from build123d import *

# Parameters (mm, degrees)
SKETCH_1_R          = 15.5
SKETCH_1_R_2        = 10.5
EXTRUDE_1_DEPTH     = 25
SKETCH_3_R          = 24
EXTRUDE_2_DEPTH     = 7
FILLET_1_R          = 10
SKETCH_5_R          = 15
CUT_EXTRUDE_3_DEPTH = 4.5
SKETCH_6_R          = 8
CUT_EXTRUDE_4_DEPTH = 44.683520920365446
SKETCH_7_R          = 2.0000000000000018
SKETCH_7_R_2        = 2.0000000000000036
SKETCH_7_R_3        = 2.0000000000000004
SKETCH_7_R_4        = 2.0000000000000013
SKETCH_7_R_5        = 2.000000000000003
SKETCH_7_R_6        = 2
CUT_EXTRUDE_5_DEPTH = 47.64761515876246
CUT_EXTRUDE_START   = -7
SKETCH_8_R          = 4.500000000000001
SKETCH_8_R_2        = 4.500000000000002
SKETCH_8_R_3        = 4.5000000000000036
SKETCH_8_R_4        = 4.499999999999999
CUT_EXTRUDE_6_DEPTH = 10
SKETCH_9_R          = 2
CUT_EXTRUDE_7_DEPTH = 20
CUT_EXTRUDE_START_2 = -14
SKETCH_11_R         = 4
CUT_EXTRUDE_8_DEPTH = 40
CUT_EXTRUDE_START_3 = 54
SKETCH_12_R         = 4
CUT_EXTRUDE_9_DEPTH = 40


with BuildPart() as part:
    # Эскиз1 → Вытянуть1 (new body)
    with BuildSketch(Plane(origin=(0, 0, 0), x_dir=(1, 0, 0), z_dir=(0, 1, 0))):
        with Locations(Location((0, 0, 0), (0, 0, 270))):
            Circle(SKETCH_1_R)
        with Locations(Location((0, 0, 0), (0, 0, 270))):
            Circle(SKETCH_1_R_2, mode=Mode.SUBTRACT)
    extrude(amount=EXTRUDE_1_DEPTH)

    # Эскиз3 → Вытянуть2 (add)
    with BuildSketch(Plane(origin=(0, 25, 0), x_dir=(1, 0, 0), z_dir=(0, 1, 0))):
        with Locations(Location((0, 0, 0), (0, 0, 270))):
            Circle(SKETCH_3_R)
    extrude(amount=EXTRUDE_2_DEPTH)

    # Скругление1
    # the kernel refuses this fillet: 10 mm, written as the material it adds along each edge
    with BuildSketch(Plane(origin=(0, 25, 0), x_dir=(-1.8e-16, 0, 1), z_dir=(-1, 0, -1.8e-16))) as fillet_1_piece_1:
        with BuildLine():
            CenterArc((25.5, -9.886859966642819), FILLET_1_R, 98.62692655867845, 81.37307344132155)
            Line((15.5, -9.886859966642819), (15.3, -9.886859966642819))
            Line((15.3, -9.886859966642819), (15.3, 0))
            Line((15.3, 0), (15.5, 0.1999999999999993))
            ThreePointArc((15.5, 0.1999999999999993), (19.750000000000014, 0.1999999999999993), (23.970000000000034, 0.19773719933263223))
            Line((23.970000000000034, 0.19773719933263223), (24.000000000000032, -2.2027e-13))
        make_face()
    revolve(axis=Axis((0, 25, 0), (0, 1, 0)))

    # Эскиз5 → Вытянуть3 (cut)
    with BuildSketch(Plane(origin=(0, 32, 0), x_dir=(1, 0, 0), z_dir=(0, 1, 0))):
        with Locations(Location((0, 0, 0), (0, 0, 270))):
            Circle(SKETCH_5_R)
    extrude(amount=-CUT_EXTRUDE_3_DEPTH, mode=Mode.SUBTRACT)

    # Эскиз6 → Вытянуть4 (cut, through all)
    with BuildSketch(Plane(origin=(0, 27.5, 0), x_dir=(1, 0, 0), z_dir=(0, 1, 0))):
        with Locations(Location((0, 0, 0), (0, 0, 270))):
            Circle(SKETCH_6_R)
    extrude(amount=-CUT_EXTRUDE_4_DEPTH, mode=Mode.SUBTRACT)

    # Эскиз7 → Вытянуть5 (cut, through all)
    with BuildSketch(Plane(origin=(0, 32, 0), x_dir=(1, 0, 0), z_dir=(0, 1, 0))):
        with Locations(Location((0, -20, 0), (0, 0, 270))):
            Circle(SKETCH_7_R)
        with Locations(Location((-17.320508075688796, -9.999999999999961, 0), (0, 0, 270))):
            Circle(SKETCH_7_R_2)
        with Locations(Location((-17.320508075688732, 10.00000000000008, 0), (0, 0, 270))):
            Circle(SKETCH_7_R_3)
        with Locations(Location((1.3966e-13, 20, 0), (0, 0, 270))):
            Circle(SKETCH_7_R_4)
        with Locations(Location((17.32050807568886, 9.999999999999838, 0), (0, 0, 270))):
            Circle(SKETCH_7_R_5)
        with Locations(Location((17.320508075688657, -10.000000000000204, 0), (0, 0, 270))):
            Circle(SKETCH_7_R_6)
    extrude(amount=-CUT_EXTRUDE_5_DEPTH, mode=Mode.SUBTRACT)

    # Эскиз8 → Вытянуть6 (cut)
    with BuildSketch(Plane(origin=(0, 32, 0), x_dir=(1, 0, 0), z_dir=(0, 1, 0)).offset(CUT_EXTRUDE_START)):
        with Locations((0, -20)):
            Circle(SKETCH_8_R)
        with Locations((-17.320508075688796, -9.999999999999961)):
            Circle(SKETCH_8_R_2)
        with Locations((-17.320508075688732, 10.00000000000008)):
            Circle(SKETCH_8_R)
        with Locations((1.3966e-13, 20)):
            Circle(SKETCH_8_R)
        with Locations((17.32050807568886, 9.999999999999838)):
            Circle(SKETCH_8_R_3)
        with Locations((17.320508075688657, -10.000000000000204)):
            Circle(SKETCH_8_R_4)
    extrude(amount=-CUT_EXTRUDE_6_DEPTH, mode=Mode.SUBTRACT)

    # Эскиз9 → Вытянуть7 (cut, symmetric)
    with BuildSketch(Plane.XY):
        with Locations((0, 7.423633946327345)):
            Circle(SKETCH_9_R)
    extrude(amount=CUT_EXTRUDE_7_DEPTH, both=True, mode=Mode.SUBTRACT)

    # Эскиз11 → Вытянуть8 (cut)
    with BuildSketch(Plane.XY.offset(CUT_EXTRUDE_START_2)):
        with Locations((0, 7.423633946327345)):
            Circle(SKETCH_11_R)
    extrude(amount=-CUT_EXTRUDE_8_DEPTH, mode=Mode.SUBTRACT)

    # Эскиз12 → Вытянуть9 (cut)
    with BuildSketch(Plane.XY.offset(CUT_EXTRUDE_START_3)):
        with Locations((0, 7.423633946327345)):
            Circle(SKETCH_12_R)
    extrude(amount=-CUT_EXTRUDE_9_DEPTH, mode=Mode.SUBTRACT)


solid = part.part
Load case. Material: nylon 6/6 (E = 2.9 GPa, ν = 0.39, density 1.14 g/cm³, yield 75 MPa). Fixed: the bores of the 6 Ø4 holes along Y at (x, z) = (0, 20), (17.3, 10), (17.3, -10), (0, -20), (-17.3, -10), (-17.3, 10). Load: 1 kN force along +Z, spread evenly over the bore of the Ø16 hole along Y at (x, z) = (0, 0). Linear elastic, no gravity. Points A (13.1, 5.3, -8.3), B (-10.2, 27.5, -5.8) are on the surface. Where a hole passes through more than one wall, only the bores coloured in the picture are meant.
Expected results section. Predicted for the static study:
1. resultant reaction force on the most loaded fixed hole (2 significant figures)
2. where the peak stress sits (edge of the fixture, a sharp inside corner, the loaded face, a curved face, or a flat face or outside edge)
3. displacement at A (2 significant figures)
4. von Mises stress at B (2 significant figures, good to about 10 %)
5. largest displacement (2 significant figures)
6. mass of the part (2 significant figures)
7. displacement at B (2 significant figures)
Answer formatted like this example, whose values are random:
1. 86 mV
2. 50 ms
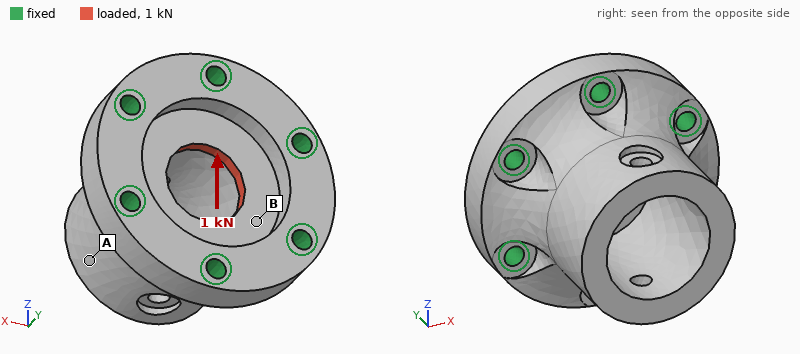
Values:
1. 230 N
2. a sharp inside corner
3. 6.0 µm
4. 5.2 MPa
5. 30 µm
6. 23 g
7. 14 µm
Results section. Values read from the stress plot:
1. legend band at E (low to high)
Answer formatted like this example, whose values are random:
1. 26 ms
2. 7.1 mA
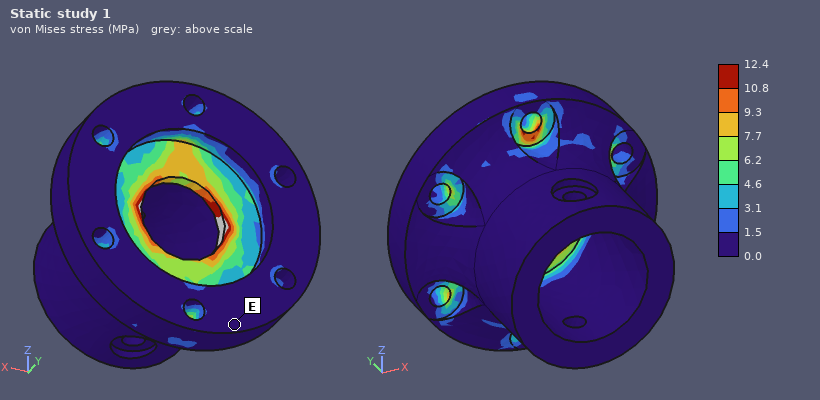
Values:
1. 0.0 to 1.5 MPa
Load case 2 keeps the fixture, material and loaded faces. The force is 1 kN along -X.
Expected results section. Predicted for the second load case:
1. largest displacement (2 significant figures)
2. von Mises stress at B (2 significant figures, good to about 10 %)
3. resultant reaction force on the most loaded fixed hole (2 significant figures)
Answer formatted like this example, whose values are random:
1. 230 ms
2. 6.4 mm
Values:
1. 31 µm
2. 8.0 MPa
3. 210 N
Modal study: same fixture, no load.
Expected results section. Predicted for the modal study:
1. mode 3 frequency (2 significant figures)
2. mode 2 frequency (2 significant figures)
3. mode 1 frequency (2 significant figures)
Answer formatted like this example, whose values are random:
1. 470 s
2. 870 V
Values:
1. 7300 Hz
2. 6000 Hz
3. 5900 Hz
